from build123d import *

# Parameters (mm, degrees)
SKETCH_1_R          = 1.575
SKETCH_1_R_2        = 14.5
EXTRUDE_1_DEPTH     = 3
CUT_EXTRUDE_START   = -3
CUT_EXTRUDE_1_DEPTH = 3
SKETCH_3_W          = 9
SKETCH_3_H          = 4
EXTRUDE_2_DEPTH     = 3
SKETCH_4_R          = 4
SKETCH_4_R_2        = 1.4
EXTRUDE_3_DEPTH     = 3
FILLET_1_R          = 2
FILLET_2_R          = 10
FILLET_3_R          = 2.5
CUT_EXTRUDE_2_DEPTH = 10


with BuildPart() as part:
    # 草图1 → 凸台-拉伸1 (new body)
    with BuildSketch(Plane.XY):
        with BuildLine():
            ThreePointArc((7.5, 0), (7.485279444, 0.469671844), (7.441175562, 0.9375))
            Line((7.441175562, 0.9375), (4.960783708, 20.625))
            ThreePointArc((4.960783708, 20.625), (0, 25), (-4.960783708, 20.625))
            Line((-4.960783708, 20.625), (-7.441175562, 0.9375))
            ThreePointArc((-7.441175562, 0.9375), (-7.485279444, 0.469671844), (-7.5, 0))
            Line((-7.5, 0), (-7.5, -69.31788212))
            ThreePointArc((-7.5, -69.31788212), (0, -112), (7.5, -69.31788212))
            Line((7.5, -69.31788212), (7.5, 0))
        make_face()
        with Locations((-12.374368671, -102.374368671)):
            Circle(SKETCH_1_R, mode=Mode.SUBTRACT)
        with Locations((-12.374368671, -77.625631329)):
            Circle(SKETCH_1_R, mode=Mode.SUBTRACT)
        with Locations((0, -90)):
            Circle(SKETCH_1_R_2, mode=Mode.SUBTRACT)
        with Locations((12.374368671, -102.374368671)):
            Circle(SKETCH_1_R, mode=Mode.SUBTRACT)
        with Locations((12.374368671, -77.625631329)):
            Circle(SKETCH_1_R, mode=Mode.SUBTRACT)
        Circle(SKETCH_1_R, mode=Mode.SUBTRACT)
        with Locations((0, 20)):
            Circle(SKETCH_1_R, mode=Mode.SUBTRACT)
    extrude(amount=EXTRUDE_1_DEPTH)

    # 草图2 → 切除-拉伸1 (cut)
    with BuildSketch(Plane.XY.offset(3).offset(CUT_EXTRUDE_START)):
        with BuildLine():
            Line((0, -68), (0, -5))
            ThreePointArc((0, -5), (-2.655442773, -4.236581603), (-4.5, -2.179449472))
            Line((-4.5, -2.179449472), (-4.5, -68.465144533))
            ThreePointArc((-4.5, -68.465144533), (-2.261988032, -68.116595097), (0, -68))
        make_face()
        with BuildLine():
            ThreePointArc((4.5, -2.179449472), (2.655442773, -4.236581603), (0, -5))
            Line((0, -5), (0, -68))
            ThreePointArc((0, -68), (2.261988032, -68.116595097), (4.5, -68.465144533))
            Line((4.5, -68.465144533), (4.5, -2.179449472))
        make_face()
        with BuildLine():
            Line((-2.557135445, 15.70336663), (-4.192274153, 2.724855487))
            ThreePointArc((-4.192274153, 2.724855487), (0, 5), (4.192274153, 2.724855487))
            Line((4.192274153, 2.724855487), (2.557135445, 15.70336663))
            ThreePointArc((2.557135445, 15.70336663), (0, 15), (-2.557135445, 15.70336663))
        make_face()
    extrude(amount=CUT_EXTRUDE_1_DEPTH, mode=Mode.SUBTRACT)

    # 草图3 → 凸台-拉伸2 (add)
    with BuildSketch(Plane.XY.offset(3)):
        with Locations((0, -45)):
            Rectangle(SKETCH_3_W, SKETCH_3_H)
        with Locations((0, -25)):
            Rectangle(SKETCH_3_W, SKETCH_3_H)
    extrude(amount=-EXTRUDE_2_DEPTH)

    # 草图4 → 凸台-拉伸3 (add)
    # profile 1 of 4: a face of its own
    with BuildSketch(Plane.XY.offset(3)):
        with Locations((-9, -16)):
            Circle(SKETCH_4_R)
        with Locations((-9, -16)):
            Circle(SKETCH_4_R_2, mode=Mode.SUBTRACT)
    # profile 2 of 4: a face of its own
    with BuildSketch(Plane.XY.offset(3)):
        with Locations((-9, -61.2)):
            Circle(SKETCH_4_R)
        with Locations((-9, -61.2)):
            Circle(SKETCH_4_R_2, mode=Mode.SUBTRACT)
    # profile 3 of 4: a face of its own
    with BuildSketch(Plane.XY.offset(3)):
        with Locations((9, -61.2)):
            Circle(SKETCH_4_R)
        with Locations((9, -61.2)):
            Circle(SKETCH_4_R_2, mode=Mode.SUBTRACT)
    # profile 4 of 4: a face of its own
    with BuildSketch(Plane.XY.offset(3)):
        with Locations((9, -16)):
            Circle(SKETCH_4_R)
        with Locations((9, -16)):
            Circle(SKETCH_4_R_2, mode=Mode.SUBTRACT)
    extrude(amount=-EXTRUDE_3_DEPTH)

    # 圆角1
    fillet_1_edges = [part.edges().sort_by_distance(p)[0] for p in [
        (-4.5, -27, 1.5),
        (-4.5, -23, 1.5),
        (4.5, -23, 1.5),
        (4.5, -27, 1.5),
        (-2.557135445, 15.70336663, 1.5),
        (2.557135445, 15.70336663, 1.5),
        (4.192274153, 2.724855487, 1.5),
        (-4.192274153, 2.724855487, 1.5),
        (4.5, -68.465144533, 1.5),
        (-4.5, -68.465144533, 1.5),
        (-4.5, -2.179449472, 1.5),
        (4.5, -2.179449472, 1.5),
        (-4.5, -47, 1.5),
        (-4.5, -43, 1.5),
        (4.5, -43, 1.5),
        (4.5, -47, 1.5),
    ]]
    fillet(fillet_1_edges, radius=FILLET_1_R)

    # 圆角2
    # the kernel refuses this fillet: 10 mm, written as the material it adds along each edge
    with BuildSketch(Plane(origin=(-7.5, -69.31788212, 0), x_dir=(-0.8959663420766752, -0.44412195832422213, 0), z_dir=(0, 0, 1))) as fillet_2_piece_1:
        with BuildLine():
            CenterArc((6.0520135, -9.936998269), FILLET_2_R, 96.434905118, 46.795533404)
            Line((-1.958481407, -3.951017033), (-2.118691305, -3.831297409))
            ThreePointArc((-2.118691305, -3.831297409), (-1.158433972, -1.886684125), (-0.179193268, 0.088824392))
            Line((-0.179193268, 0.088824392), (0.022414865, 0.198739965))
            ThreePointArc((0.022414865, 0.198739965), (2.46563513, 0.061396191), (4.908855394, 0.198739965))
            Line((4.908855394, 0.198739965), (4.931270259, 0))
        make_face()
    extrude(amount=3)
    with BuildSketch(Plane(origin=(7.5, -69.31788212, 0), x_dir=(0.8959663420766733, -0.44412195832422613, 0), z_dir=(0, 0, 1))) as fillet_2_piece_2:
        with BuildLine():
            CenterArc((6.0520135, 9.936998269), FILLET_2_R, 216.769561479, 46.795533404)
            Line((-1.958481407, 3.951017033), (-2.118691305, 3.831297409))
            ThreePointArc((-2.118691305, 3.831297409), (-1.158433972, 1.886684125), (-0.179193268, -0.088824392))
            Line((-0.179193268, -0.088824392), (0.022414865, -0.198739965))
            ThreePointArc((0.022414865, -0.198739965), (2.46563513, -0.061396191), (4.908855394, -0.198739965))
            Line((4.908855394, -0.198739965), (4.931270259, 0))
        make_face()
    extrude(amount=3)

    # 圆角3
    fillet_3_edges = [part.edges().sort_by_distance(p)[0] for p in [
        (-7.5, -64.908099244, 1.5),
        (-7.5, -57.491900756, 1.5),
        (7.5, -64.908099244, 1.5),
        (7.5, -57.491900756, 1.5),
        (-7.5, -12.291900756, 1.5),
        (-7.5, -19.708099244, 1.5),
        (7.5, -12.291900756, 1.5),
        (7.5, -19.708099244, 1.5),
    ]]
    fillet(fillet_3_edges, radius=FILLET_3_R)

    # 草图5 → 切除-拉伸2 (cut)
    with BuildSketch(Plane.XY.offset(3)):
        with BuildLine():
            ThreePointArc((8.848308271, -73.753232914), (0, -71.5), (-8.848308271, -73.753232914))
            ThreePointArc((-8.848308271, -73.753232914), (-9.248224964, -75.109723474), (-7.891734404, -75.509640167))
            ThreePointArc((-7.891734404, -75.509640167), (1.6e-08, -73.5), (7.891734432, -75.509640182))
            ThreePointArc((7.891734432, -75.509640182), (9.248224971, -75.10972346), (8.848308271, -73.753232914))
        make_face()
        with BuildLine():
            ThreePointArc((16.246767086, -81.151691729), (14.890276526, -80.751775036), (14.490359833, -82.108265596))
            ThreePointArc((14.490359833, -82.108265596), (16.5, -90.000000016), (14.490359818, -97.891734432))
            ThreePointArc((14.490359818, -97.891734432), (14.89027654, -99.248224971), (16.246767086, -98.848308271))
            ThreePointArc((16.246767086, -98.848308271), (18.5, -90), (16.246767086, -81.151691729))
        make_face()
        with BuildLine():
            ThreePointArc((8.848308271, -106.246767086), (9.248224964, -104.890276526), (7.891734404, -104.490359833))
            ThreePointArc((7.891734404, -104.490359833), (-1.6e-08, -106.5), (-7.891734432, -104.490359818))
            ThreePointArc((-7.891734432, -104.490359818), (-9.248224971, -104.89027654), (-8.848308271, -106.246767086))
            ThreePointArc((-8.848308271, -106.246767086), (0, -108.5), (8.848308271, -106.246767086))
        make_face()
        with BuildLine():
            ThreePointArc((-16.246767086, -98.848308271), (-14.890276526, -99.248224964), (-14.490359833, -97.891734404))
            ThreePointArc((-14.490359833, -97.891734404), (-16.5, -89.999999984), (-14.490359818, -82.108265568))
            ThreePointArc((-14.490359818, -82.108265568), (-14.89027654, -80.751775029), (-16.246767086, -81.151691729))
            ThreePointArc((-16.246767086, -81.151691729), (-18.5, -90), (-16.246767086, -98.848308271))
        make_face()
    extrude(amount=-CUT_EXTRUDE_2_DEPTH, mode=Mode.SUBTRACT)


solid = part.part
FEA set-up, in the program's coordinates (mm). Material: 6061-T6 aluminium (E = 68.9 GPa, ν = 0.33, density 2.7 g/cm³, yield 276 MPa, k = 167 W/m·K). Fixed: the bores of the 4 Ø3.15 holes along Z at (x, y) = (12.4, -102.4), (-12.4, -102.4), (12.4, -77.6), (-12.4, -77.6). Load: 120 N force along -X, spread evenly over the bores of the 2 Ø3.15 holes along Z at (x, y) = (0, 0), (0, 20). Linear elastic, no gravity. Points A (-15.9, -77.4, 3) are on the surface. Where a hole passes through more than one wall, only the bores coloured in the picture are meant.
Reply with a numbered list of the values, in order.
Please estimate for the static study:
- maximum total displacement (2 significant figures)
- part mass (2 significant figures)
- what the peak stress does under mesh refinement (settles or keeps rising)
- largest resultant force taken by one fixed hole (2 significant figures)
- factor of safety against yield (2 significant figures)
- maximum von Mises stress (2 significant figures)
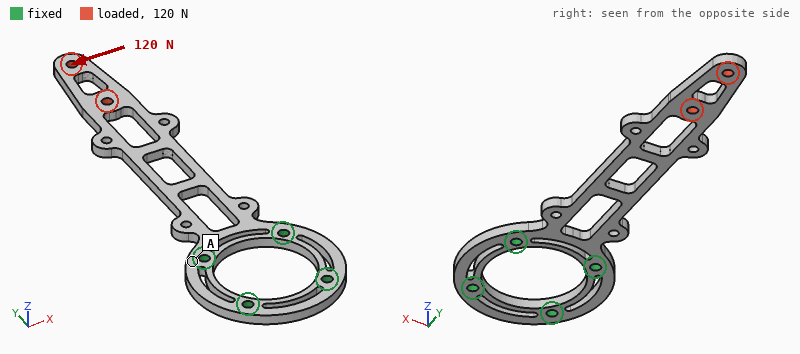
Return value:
1. 0.75 mm
2. 13 g
3. settles
4. 500 N
5. 1.6
6. 180 MPa
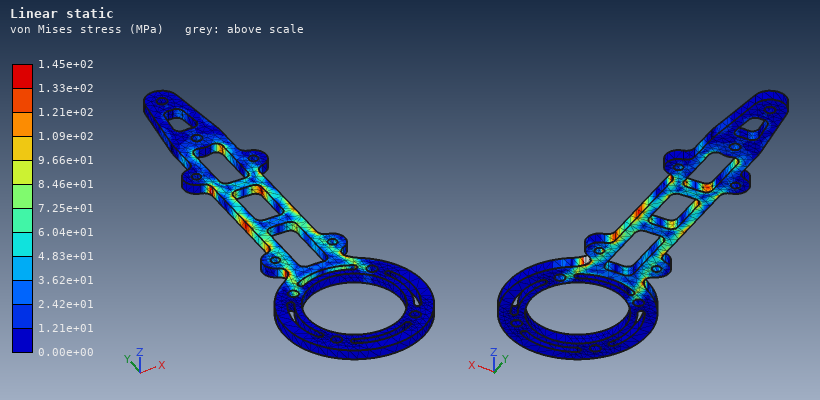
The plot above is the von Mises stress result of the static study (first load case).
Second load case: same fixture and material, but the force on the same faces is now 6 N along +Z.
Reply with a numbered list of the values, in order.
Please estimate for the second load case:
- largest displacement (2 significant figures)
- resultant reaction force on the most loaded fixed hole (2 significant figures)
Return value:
1. 1.5 mm
2. 3.2 N
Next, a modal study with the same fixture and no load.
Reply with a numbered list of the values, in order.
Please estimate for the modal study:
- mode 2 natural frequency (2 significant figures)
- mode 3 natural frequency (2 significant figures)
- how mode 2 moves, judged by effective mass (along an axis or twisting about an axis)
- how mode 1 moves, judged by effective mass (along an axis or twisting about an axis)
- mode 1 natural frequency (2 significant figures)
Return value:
1. 1300 Hz
2. 1300 Hz
3. along X
4. along Z
5. 210 Hz
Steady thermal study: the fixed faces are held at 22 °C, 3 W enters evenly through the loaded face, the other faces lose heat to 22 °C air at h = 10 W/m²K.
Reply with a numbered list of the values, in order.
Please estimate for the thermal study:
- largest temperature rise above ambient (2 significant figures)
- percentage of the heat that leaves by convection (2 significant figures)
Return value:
1. 54 K
2. 31 %
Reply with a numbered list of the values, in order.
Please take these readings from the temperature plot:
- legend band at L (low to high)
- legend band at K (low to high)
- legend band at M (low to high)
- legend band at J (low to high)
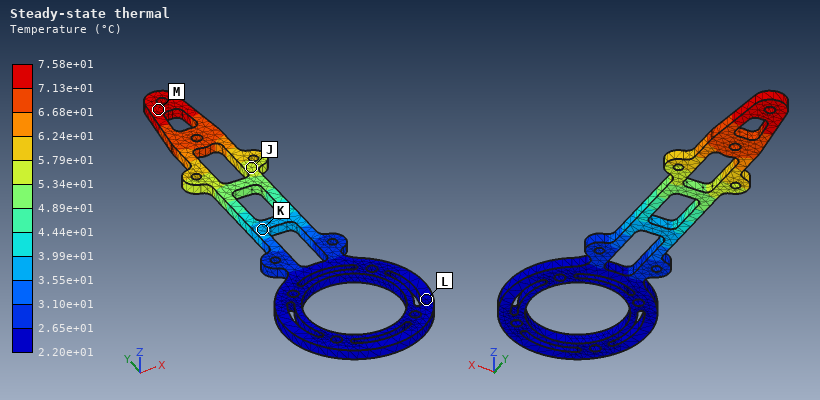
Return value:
1. 2.20e+01 to 2.65e+01 °C
2. 3.55e+01 to 3.99e+01 °C
3. 7.13e+01 to 7.58e+01 °C
4. 5.34e+01 to 5.79e+01 °C
